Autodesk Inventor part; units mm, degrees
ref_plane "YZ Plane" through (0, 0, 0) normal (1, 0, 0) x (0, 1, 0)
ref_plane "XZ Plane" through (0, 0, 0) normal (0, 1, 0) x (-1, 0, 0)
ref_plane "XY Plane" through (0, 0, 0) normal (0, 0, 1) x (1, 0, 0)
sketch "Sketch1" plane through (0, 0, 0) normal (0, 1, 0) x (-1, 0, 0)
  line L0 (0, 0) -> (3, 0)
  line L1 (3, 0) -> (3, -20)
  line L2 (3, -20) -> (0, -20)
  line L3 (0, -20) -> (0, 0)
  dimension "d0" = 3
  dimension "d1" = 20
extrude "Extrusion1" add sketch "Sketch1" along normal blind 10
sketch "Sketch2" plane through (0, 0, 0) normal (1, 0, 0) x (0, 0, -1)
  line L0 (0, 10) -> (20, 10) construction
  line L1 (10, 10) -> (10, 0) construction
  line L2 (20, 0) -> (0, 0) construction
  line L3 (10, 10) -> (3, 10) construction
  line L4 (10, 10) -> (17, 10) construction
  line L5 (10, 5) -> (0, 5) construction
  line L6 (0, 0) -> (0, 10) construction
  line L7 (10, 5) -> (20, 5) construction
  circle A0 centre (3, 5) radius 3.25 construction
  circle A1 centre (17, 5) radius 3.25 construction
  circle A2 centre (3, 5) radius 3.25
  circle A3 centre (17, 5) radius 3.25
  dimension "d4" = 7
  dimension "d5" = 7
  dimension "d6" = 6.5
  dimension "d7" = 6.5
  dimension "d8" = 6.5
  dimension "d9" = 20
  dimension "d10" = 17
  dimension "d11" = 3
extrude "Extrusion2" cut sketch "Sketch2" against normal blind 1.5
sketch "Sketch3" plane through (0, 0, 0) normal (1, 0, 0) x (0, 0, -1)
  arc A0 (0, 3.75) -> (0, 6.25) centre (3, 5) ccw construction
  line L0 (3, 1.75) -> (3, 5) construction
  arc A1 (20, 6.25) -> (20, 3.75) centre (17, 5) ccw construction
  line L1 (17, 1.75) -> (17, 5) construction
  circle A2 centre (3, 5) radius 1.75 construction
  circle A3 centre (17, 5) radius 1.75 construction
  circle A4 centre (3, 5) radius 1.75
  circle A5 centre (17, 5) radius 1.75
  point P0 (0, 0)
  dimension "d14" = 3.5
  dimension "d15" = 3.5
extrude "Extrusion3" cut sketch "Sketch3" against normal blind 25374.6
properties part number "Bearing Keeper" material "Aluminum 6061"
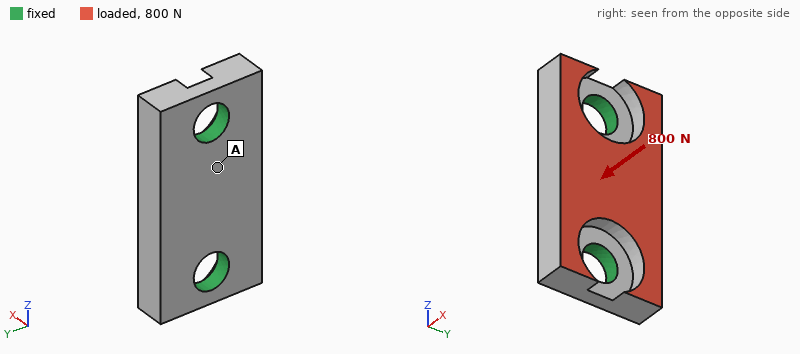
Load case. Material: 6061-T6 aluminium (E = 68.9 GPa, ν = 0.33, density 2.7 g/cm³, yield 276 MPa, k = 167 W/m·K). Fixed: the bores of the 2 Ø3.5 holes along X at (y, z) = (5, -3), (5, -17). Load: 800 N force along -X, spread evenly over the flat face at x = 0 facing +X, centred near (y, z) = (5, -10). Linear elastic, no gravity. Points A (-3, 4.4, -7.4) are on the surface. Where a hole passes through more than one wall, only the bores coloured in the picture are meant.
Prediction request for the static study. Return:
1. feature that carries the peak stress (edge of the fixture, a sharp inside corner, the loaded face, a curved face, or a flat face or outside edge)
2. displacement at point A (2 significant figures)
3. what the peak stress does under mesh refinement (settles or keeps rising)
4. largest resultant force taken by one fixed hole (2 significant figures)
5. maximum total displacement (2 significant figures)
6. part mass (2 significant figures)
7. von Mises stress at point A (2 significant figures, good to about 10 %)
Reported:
edge of the fixture
5.7 µm
keeps rising
430 N
9.9 µm
1.3 g
31 MPa
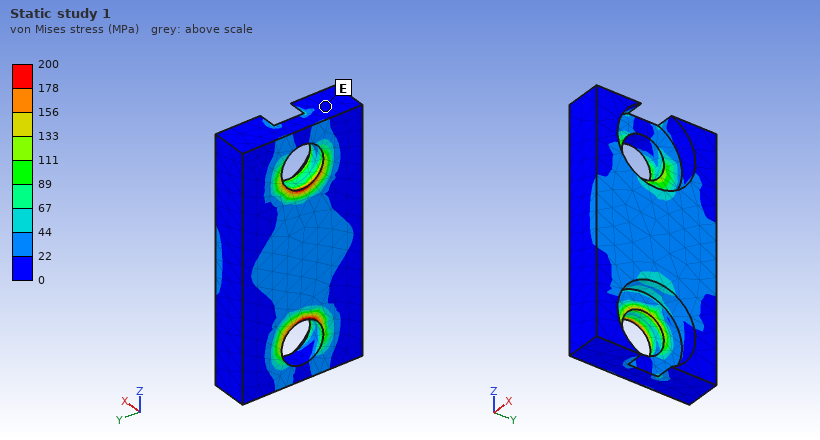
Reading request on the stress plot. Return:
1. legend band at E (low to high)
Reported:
0 to 22 MPa
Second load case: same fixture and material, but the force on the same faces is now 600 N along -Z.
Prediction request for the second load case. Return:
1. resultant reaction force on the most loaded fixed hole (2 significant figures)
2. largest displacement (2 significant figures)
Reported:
320 N
3.7 µm
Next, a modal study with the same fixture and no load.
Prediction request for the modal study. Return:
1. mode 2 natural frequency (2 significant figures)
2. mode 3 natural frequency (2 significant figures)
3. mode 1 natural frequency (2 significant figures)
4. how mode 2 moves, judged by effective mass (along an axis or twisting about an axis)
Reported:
51 kHz
70 kHz
39 kHz
along X
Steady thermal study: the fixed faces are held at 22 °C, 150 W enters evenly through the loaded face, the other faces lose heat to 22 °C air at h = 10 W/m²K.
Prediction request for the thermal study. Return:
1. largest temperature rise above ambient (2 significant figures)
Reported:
82 K
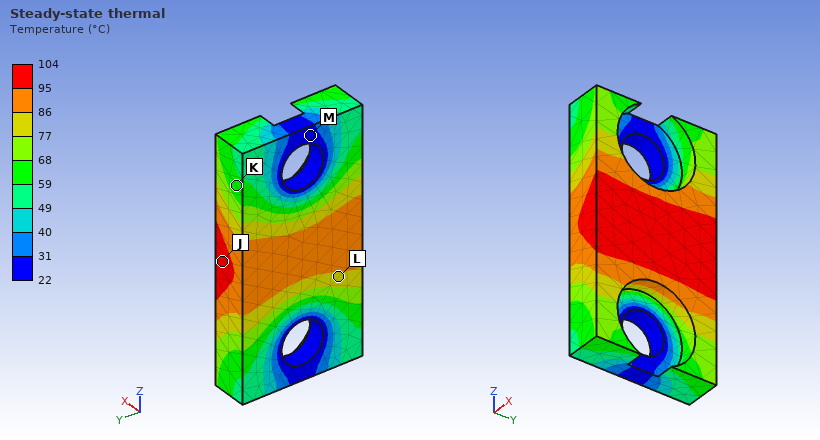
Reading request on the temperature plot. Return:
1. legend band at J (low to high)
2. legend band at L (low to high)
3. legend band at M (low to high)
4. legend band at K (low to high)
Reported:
95 to 104 °C
77 to 86 °C
22 to 31 °C
59 to 68 °C
